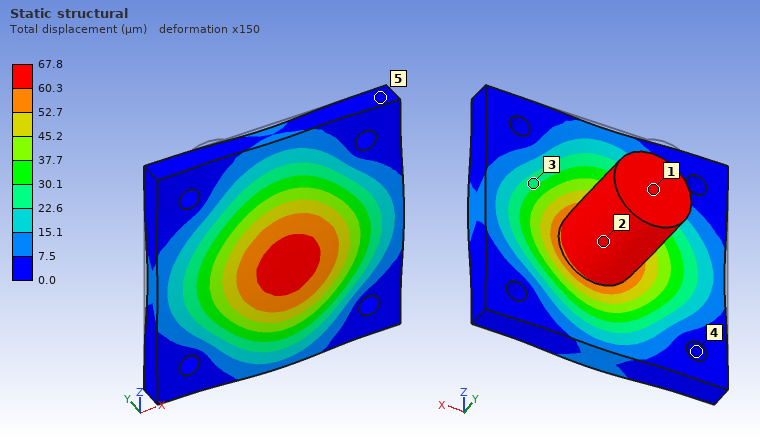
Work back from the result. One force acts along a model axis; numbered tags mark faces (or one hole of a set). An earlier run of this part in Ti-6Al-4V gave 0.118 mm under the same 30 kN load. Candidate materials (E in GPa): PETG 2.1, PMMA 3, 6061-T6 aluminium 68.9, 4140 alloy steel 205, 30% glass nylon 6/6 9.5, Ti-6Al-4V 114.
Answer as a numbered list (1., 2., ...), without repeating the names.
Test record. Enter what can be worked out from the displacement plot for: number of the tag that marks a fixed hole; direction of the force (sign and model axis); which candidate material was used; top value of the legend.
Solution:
1. 4
2. -Y
3. 4140 alloy steel
4. 67.8 µm
